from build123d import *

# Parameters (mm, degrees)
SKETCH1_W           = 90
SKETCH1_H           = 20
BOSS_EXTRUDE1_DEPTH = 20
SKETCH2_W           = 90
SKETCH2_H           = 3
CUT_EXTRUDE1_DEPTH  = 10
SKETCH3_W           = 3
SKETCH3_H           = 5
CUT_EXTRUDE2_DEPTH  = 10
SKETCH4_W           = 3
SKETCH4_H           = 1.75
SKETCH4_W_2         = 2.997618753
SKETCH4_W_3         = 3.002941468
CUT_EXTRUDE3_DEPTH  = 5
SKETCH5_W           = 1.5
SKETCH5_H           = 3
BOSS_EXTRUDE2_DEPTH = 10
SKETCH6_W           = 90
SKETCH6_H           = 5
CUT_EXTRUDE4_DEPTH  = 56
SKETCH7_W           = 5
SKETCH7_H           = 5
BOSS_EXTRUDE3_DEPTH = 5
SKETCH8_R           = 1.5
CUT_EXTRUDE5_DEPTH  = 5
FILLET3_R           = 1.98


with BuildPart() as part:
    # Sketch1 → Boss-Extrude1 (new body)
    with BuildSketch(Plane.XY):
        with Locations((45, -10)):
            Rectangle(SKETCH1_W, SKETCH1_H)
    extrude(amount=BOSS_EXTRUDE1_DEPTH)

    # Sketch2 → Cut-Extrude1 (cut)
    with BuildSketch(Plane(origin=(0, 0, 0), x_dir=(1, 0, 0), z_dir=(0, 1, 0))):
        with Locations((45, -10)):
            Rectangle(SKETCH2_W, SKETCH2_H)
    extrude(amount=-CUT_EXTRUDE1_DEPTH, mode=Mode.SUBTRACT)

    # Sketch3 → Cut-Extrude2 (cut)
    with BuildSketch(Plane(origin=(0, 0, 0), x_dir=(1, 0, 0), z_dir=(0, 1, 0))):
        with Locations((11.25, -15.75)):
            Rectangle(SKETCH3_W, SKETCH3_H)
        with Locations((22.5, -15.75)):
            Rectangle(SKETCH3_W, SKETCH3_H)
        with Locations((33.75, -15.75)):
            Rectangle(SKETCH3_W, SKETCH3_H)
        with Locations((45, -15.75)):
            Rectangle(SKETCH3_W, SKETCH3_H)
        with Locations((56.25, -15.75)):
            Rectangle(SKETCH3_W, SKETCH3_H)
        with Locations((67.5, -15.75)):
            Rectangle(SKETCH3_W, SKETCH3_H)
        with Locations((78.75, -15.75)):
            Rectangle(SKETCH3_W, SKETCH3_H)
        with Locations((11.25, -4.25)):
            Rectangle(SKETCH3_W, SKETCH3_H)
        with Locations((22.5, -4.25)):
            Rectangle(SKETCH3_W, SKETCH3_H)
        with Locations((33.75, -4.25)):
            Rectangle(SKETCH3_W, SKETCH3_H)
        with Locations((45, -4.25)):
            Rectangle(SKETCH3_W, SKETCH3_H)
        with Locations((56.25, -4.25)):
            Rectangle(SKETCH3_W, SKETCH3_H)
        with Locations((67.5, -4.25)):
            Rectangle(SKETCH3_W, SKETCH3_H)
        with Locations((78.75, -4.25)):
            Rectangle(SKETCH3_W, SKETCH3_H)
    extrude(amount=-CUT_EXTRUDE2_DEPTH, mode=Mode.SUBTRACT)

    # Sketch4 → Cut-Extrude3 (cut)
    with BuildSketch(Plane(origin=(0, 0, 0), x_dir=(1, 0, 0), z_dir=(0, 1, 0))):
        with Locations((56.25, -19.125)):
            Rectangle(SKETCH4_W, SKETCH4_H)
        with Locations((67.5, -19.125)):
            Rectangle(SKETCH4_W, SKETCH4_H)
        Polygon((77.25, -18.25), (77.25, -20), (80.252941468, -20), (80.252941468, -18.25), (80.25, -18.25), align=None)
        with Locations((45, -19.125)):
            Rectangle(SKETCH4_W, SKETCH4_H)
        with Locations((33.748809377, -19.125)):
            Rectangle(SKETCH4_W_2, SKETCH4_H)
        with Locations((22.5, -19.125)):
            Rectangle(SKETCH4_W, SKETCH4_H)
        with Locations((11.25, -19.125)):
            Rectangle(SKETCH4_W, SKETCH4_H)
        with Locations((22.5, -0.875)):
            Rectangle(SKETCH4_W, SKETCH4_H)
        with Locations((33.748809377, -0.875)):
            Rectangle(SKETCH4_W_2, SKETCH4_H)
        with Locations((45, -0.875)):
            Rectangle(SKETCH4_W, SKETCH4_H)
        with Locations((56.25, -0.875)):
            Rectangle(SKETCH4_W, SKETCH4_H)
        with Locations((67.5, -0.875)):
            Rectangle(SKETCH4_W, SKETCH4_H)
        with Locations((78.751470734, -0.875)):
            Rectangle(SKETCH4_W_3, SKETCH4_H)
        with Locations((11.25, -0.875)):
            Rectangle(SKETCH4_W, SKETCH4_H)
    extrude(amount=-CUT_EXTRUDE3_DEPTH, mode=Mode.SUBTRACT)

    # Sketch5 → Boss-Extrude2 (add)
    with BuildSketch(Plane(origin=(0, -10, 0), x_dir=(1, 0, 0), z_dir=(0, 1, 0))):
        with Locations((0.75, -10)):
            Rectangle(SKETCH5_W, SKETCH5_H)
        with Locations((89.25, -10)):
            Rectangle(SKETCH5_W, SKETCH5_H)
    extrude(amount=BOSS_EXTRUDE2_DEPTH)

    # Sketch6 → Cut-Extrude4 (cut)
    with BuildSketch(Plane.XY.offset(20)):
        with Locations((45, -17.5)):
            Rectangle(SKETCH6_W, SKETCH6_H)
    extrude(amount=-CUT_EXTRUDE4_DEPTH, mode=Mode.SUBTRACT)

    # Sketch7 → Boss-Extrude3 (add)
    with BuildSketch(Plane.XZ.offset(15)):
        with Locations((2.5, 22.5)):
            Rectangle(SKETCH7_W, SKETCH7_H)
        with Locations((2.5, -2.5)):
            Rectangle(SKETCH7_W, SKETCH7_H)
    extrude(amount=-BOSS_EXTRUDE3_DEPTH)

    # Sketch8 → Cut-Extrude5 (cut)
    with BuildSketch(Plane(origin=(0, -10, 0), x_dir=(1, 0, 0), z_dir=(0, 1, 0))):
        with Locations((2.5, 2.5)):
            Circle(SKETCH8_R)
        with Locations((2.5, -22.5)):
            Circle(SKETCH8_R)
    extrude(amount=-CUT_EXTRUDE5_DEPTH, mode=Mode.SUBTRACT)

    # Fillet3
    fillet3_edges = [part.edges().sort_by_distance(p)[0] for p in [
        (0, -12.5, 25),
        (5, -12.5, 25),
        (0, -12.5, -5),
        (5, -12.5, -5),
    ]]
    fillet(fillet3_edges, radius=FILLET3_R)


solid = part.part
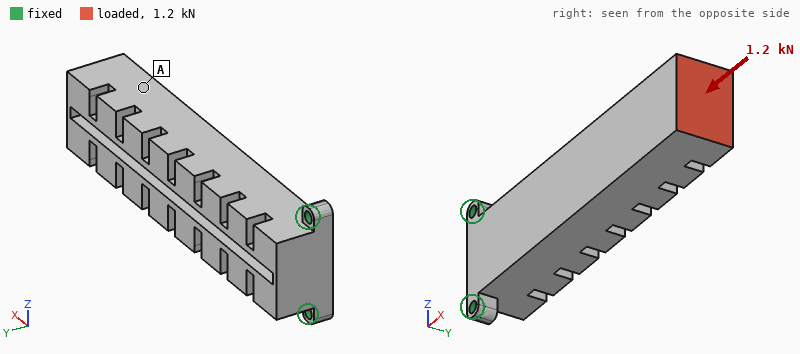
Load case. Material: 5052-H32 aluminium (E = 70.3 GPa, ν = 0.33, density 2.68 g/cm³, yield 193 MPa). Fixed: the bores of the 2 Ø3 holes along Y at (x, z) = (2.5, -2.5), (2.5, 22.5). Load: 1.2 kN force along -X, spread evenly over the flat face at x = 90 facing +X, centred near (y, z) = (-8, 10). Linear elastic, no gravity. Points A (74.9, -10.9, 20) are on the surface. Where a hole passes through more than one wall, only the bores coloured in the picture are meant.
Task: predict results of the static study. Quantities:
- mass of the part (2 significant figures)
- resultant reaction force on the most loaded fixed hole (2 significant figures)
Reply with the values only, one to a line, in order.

59 g
640 N
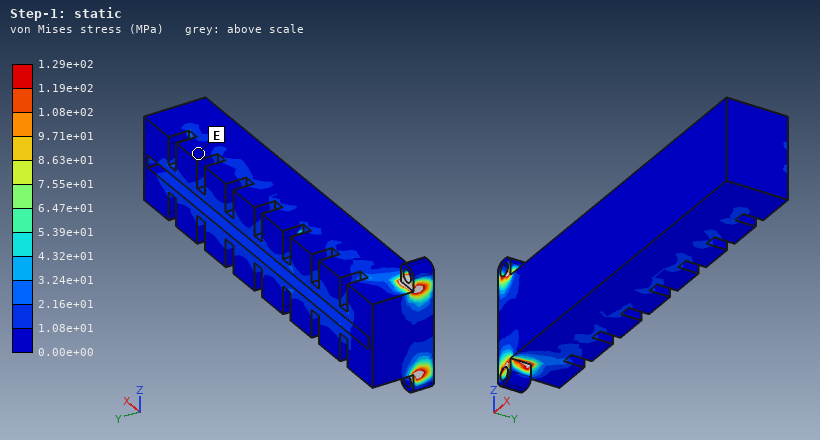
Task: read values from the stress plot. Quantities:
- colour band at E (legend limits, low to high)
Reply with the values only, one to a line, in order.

0.00e+00 to 1.08e+01 MPa
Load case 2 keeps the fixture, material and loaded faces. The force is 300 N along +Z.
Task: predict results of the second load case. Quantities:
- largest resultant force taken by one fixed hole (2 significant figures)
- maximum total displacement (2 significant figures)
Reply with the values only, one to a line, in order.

1.2 kN
0.25 mm
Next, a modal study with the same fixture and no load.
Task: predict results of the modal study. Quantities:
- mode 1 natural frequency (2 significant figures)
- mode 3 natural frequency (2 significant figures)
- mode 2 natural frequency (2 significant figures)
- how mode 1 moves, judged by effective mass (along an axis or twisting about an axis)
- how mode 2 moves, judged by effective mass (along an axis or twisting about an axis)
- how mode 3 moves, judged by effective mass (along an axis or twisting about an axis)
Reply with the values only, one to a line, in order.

490 Hz
4400 Hz
1400 Hz
along Y
along Z
twisting about X
